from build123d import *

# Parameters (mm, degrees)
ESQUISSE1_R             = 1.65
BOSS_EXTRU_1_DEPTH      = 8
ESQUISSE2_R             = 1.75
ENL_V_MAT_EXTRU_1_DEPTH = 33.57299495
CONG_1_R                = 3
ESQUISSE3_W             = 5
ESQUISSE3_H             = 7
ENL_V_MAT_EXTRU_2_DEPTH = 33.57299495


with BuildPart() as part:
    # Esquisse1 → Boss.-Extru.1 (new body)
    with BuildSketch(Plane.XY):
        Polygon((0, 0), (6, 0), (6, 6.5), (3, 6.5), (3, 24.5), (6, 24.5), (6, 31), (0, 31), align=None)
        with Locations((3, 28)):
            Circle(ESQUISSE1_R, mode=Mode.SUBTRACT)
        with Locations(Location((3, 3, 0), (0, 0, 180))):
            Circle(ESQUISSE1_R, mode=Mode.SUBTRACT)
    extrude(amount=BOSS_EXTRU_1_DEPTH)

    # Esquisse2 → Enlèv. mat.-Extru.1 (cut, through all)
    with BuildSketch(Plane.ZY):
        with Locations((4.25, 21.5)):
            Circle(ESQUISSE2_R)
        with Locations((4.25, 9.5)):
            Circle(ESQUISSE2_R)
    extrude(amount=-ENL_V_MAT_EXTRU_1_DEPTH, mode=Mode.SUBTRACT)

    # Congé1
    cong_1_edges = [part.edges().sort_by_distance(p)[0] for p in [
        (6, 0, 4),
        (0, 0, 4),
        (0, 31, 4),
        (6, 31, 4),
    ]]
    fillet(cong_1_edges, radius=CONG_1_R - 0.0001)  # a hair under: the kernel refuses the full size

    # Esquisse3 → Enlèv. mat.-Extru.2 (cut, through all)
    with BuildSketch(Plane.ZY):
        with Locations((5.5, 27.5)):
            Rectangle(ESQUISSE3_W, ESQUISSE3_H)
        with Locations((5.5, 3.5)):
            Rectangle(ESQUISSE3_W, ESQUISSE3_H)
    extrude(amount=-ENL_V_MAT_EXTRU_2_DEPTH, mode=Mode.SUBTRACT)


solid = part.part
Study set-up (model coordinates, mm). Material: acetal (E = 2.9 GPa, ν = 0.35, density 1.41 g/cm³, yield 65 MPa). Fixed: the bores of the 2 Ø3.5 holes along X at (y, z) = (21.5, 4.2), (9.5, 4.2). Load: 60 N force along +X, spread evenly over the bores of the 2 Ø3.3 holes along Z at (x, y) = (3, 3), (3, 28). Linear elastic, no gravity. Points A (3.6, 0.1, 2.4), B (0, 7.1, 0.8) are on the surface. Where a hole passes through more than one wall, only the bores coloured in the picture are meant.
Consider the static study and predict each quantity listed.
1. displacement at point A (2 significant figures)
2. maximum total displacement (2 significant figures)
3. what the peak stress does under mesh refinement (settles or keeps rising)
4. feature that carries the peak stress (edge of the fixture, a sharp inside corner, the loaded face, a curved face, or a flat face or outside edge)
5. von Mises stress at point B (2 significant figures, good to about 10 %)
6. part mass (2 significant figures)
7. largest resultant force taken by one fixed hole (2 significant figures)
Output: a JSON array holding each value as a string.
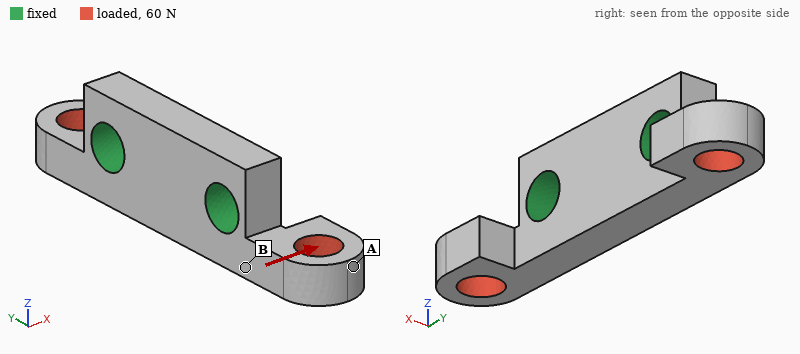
["0.22 mm", "0.22 mm", "keeps rising", "a sharp inside corner", "20 MPa", "0.73 g", "30 N"]
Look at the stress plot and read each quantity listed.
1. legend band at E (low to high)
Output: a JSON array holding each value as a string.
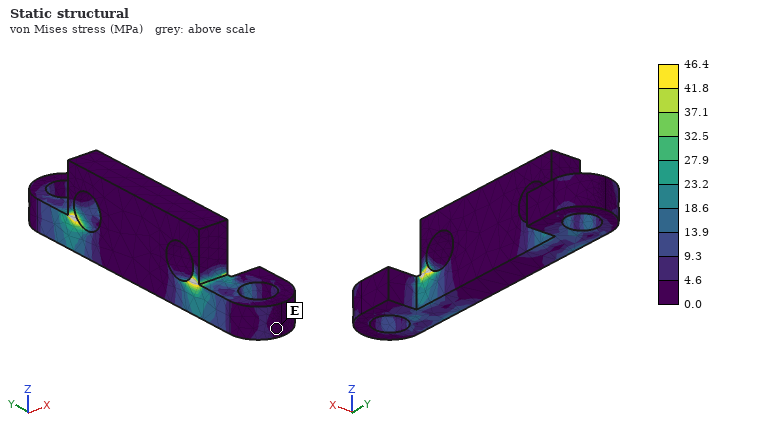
["0.0 to 4.6 MPa"]
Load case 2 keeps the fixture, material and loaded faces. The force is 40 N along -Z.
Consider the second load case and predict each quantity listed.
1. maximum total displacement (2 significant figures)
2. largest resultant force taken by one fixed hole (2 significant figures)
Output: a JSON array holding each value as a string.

["0.14 mm", "24 N"]
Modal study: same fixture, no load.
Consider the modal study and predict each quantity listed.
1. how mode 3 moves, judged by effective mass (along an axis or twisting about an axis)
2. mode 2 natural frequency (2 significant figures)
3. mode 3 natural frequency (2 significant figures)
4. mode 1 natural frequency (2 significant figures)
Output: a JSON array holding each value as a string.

["twisting about X", "6700 Hz", "7600 Hz", "6700 Hz"]
